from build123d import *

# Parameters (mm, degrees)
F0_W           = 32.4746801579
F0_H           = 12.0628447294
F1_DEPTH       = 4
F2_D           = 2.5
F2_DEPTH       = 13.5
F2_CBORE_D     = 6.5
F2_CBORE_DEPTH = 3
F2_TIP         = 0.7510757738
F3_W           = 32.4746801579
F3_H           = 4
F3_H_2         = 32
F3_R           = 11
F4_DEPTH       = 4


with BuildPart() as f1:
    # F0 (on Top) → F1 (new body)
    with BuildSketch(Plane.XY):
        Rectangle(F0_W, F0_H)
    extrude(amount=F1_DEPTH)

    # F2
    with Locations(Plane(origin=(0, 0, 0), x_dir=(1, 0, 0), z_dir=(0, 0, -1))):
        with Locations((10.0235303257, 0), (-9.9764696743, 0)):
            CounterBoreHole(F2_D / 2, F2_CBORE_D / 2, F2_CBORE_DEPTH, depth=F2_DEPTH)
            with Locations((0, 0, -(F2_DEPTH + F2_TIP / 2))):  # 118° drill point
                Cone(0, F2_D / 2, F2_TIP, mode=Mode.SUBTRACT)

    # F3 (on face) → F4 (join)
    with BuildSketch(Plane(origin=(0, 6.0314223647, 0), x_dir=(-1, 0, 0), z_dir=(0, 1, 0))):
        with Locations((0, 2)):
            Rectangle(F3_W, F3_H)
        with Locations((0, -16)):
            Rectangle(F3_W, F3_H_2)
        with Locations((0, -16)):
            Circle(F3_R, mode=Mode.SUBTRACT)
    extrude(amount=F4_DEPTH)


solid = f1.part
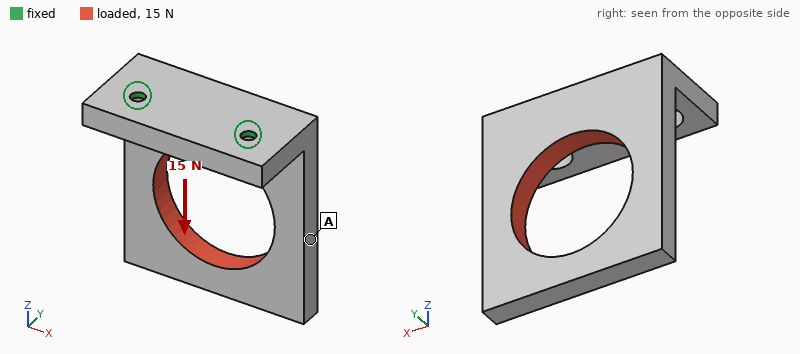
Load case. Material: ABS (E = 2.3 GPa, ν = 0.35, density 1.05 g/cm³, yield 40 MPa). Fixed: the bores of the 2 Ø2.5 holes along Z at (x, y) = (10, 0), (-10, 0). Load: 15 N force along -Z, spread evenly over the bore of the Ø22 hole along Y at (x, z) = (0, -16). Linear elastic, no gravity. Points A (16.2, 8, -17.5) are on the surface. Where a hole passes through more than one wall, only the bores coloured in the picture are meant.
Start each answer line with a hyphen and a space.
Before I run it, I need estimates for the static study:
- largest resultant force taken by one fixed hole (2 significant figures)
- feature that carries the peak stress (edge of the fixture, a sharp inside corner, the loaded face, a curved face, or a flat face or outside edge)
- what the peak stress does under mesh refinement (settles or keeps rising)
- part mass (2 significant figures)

- 7.5 N
- edge of the fixture
- keeps rising
- 4.7 g
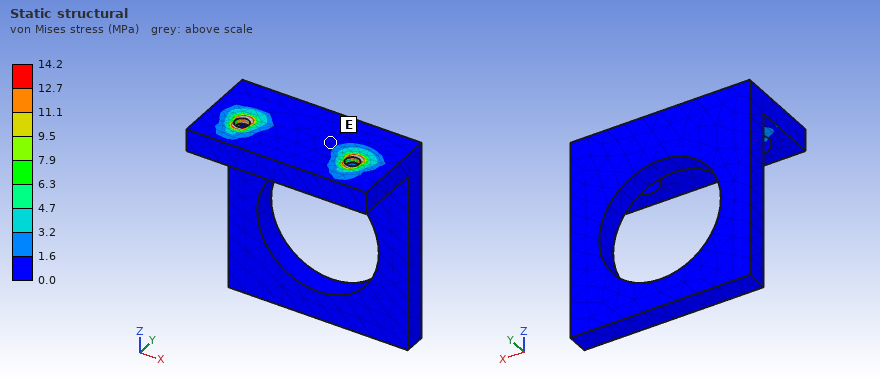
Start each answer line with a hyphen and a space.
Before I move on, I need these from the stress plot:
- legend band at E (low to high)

- 0.0 to 1.6 MPa
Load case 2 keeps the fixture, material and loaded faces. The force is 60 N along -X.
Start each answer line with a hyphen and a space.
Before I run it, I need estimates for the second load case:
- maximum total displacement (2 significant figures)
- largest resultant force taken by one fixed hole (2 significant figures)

- 0.52 mm
- 68 N
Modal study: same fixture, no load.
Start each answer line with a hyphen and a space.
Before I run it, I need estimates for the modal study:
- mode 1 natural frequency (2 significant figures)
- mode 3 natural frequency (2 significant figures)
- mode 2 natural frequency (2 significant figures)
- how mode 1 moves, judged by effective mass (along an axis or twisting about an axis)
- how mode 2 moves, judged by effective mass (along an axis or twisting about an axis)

- 330 Hz
- 1500 Hz
- 1100 Hz
- along Y
- along X
